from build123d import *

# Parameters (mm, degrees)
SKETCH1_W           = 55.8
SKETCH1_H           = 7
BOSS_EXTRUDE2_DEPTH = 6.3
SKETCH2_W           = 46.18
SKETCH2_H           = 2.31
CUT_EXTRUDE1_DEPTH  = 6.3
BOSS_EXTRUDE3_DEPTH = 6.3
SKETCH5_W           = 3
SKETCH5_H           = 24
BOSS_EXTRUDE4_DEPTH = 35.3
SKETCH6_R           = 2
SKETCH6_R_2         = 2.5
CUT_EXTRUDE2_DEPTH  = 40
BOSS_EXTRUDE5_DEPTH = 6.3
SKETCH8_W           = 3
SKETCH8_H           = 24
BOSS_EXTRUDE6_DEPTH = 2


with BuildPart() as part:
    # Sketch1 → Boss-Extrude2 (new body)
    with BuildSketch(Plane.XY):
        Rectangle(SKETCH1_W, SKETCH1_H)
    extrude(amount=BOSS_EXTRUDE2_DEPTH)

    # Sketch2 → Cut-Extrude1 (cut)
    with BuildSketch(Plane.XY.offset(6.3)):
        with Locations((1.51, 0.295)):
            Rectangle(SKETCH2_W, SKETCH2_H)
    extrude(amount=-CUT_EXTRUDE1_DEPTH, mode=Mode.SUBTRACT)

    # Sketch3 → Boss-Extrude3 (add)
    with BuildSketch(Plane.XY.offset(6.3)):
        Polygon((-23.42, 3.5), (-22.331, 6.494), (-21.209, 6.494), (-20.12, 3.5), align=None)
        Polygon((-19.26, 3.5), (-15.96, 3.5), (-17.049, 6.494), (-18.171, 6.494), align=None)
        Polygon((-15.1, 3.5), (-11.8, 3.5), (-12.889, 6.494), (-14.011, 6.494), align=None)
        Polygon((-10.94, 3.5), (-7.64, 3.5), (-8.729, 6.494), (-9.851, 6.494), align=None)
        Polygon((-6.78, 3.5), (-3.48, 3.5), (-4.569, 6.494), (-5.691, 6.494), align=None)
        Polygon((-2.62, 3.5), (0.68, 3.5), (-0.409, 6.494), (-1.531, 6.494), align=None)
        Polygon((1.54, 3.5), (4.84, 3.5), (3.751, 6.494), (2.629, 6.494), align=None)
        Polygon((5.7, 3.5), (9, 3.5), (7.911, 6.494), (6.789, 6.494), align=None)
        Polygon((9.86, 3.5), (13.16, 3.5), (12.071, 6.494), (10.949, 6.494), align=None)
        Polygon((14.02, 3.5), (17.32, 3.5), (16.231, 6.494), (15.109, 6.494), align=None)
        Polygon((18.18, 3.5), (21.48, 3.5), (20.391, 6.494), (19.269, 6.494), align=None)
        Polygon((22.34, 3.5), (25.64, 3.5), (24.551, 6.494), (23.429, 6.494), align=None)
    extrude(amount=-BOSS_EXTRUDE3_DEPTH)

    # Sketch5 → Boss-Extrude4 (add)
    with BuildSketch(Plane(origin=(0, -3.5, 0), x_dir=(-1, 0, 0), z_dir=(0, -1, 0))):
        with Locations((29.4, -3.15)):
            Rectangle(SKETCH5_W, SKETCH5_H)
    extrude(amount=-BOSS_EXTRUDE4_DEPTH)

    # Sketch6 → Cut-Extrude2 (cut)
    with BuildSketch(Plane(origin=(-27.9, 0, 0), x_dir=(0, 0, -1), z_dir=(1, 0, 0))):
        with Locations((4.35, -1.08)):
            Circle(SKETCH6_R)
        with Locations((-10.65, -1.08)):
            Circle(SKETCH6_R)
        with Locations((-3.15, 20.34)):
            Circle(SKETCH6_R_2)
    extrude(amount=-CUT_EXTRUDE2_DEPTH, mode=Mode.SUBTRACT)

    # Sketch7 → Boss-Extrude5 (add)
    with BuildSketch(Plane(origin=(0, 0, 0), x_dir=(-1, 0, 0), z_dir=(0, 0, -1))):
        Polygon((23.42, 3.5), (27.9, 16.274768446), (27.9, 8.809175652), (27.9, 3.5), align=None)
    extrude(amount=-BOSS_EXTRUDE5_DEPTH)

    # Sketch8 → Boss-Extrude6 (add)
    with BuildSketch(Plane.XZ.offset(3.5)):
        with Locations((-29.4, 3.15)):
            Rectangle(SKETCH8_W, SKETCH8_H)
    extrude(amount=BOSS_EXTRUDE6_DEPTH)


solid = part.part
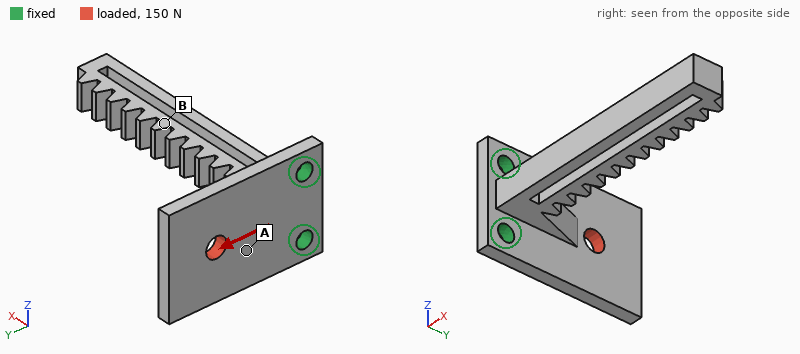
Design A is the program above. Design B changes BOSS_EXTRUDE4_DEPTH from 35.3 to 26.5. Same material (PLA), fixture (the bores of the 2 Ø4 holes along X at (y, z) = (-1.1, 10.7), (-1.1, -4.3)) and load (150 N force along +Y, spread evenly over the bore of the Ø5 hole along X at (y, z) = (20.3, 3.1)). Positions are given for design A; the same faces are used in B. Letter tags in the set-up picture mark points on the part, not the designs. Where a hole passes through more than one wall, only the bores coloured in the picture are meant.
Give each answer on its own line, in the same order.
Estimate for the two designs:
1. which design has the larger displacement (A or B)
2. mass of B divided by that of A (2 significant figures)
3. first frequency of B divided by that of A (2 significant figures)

B
0.87
1.0
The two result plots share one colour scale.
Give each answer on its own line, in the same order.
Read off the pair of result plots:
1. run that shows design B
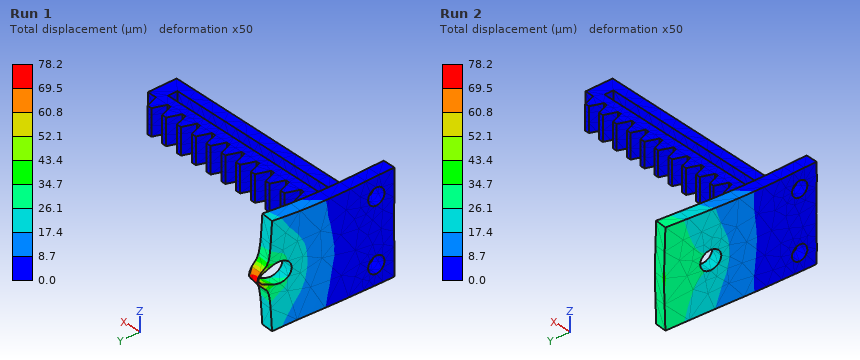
Run 1
